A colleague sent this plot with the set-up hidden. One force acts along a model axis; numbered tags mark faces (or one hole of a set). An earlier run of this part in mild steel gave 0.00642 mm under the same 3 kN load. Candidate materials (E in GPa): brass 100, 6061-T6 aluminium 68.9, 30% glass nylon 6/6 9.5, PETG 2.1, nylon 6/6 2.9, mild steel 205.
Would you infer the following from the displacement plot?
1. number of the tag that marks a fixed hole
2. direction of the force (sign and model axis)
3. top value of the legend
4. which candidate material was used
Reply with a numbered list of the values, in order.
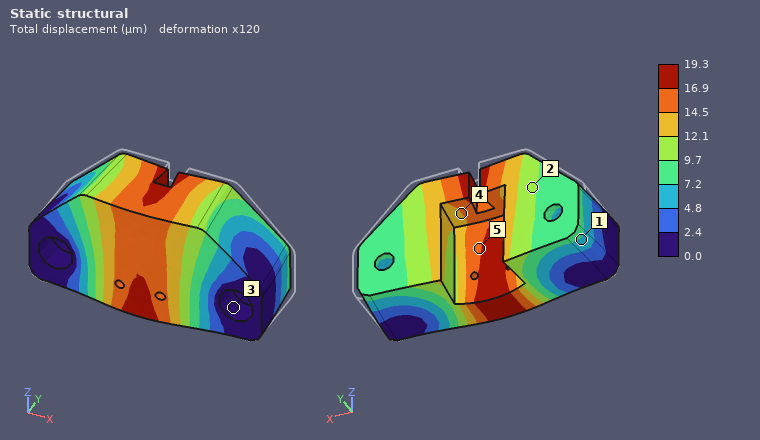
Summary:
1. 3
2. -Y
3. 19.3 µm
4. 6061-T6 aluminium
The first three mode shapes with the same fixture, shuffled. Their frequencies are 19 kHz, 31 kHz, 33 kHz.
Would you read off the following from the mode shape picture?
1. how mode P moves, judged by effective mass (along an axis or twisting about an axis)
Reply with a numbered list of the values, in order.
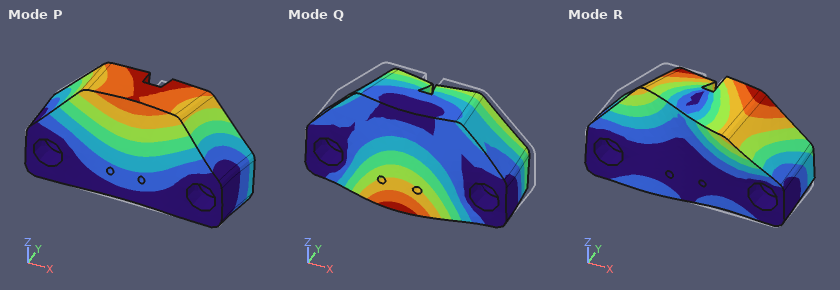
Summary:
1. along Y
